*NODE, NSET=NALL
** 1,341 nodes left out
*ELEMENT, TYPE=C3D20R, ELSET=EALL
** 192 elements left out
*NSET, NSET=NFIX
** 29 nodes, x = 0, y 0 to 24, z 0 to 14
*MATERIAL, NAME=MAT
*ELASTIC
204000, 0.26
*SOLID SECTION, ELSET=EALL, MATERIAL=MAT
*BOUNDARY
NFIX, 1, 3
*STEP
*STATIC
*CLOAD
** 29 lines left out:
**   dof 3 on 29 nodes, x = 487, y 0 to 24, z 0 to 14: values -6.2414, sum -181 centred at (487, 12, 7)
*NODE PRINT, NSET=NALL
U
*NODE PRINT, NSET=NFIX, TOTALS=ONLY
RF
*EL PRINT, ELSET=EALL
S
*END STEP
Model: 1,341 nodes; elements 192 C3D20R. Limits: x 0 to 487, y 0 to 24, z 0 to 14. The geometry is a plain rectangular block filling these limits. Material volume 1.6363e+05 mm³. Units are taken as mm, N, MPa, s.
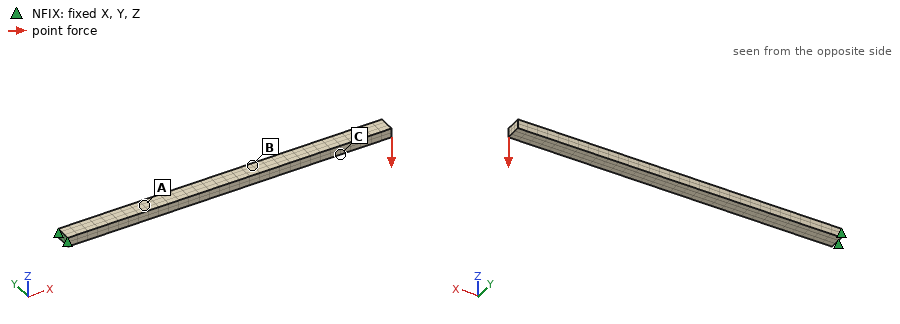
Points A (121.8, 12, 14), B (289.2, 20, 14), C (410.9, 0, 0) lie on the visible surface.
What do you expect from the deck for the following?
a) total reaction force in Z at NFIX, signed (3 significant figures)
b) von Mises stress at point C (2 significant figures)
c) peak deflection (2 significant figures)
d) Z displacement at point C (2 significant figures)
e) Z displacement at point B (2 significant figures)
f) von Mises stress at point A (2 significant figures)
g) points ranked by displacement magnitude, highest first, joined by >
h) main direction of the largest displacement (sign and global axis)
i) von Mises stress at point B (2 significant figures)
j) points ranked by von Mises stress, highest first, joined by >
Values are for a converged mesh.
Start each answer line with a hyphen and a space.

- 181 N
- 18 MPa
- 6.2 mm
- -4.8 mm
- -2.6 mm
- 84 MPa
- C > B > A
- -Z
- 46 MPa
- A > B > C
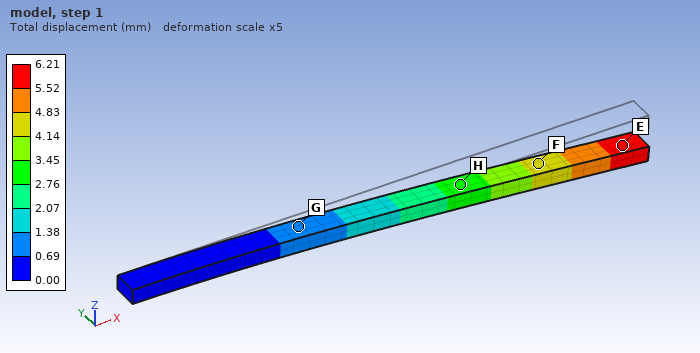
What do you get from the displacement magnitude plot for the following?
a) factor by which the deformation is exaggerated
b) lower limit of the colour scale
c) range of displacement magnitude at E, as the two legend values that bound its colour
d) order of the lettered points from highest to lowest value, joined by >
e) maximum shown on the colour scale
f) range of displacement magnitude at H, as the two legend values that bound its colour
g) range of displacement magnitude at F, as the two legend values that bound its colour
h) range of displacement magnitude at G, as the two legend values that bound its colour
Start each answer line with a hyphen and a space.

- 5
- 0.00 mm
- 5.52 to 6.21 mm
- E > F > H > G
- 6.21 mm
- 2.76 to 3.45 mm
- 4.14 to 4.83 mm
- 0.69 to 1.38 mm
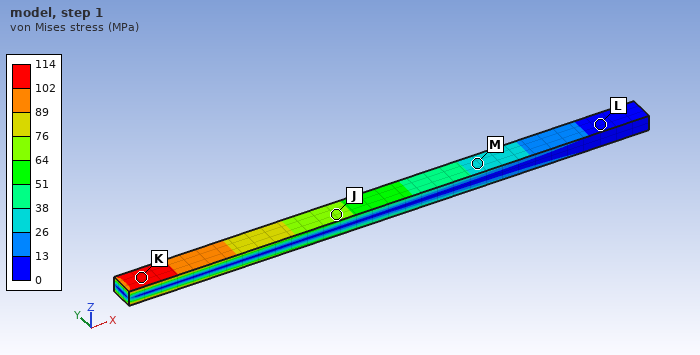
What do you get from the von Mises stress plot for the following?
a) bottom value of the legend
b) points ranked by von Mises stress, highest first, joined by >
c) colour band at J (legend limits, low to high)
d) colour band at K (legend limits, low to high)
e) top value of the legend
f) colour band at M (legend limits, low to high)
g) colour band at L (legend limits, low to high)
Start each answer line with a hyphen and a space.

- 0 MPa
- K > J > M > L
- 64 to 76 MPa
- 102 to 114 MPa
- 114 MPa
- 26 to 38 MPa
- 0 to 13 MPa
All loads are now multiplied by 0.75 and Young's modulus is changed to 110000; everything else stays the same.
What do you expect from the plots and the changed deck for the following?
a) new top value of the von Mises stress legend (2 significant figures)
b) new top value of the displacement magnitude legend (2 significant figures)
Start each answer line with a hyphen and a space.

- 86 MPa
- 8.6 mm
